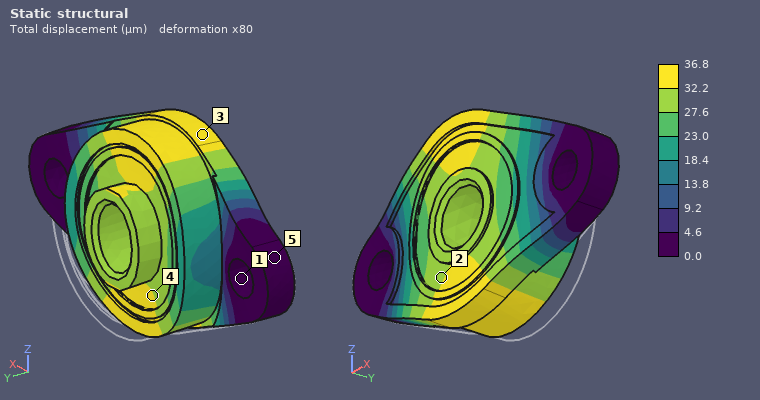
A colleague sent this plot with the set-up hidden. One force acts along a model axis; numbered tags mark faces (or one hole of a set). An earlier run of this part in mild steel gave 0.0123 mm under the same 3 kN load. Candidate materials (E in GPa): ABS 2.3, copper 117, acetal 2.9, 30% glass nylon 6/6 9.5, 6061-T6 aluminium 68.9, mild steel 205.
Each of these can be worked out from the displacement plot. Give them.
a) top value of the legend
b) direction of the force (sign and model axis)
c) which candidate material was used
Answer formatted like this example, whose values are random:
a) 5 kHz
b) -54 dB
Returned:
a) 36.8 µm
b) -Y
c) 6061-T6 aluminium
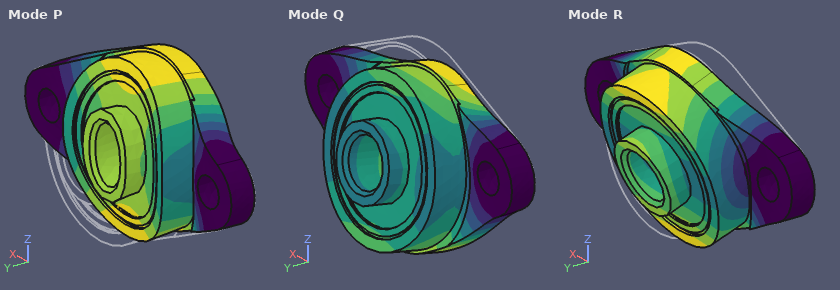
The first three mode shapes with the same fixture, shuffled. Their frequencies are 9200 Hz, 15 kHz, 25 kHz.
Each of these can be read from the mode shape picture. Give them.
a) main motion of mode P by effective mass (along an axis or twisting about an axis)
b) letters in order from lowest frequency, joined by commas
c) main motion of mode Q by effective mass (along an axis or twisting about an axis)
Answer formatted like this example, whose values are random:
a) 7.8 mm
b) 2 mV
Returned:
a) along Y
b) R, P, Q
c) along Z
